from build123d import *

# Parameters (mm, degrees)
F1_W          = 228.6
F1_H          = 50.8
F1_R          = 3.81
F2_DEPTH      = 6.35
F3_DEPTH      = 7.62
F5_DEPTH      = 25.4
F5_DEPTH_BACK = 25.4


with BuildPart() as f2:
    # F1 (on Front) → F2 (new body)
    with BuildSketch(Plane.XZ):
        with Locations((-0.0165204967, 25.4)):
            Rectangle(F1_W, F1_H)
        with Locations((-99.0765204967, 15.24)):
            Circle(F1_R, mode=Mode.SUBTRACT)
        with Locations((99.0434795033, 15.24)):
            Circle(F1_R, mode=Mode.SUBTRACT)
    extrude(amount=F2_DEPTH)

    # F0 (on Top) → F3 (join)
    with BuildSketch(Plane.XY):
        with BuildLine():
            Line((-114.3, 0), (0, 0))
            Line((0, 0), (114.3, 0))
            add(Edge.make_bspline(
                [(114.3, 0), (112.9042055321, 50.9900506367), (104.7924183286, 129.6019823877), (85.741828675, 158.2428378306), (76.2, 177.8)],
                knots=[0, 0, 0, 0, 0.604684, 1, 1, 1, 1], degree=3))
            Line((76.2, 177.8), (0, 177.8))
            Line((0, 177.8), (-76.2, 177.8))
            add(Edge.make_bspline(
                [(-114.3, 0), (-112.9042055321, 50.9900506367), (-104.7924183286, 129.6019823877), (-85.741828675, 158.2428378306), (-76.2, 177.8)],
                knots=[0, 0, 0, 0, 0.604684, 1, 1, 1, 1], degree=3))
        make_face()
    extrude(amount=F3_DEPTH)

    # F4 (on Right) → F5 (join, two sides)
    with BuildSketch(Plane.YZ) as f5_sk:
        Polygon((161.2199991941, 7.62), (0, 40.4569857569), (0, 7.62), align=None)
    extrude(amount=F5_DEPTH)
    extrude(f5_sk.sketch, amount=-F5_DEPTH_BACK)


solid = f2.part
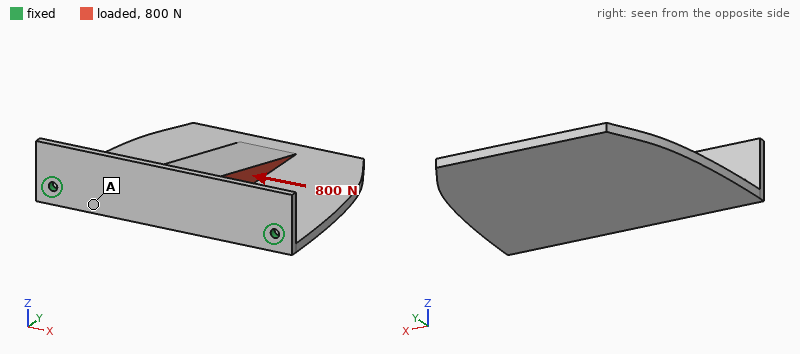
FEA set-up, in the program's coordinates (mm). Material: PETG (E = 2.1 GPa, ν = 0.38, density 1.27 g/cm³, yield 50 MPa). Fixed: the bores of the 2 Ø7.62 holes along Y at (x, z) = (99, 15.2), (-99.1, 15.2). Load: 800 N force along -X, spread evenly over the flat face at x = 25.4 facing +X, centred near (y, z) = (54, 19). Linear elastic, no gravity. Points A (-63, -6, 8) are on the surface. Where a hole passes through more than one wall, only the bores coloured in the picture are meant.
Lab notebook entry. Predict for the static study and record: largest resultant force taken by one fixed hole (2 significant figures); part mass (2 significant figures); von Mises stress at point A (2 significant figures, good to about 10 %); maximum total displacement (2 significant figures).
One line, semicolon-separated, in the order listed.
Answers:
460 N; 620 g; 0.70 MPa; 0.27 mm
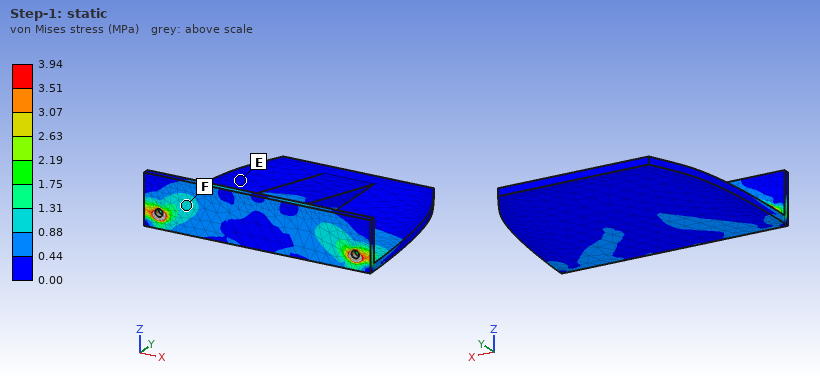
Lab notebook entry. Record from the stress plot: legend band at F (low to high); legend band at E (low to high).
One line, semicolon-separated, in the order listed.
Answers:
0.88 to 1.31 MPa; 0.00 to 0.44 MPa
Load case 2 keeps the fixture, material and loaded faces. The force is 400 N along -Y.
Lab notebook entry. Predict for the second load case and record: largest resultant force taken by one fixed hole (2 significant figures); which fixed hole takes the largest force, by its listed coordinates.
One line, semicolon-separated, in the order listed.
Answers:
270 N; (99, 15.2)
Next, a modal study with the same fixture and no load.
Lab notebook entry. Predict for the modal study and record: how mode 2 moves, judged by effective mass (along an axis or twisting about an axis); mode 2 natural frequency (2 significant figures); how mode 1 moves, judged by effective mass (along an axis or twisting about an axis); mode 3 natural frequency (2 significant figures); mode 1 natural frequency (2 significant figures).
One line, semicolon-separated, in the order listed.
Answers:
twisting about Y; 220 Hz; along Z; 350 Hz; 37 Hz
